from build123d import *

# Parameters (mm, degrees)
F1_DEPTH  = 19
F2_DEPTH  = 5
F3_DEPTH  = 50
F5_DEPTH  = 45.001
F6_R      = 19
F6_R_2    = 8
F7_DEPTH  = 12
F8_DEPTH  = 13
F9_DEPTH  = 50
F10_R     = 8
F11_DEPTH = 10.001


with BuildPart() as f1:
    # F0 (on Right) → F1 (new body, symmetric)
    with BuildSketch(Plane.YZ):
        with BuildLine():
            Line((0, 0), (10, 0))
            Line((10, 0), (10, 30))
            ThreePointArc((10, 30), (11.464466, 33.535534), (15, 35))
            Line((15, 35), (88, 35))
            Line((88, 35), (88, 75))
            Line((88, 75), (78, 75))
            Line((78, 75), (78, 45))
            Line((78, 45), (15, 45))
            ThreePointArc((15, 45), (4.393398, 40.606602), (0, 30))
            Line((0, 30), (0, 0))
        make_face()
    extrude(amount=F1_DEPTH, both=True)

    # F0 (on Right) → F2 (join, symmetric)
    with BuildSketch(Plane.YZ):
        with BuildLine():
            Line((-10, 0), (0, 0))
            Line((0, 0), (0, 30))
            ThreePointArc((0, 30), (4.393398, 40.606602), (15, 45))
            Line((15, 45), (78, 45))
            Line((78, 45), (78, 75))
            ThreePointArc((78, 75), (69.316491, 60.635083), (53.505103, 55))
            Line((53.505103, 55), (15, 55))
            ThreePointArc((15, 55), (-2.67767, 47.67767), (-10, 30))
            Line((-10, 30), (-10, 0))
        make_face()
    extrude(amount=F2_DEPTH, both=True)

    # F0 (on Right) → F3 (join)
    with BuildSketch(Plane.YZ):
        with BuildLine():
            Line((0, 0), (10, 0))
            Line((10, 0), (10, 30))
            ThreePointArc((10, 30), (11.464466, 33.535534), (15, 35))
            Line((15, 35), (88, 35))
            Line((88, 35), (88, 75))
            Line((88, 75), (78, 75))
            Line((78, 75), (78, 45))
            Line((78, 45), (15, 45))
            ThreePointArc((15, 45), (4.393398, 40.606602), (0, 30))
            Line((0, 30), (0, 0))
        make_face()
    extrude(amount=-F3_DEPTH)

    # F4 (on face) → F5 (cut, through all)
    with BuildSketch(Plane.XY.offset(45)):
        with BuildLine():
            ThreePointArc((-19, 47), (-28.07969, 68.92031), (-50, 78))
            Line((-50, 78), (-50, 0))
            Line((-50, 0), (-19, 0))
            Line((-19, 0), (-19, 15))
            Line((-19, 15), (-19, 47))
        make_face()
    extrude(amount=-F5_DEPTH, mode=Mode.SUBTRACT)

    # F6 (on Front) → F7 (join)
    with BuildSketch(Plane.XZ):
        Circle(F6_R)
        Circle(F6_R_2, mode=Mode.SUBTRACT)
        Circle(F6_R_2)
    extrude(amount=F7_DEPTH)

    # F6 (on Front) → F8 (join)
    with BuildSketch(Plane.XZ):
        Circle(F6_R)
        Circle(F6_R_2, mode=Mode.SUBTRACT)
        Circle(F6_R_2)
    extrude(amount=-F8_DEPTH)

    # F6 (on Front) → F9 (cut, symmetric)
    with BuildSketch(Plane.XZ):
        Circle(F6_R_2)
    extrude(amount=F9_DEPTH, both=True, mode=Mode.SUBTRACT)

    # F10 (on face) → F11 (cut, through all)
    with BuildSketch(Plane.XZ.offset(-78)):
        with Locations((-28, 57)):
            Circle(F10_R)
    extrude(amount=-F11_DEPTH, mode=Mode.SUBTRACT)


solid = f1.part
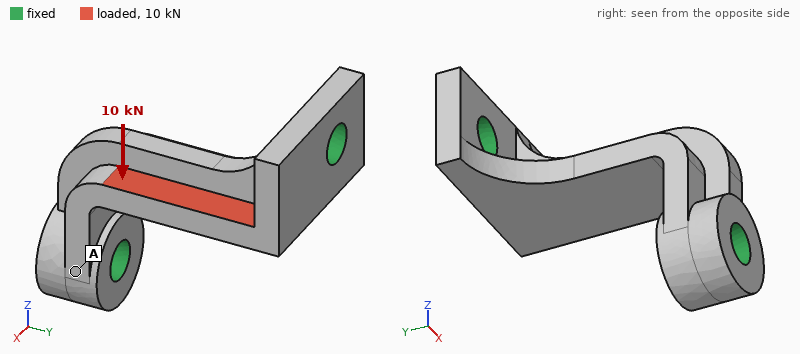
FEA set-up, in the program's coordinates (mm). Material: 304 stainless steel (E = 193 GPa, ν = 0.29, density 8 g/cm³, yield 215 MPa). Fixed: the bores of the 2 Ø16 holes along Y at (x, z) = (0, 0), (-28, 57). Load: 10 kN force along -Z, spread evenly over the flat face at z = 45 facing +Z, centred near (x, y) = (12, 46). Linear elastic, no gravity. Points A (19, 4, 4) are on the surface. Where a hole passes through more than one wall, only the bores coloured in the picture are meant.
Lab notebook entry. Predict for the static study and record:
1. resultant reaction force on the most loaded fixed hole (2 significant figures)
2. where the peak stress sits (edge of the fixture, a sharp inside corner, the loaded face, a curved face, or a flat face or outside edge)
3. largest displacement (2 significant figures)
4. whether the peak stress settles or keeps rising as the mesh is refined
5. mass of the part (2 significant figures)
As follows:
5.2 kN
edge of the fixture
60 µm
keeps rising
790 g
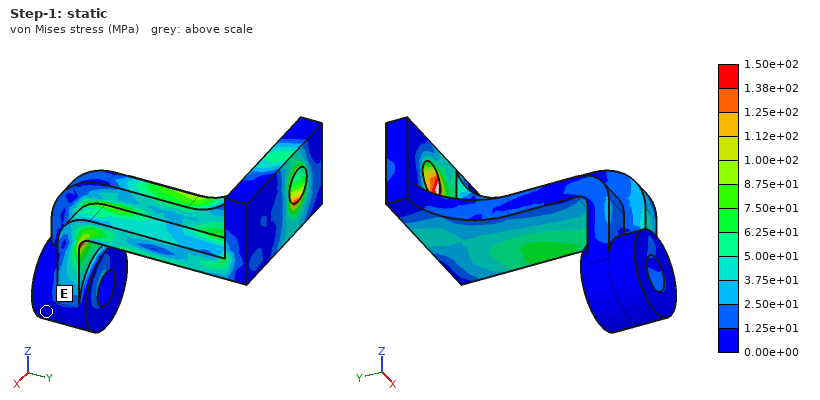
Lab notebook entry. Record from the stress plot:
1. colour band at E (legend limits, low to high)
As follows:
0.00e+00 to 1.25e+01 MPa
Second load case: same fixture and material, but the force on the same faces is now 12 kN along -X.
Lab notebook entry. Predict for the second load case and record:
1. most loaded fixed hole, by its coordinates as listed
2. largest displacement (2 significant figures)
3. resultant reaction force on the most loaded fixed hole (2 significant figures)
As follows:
(-28, 57)
32 µm
7.5 kN
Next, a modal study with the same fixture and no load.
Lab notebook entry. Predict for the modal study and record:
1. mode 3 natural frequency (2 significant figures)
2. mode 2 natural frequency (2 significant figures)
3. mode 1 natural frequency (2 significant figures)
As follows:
7900 Hz
6300 Hz
5100 Hz
